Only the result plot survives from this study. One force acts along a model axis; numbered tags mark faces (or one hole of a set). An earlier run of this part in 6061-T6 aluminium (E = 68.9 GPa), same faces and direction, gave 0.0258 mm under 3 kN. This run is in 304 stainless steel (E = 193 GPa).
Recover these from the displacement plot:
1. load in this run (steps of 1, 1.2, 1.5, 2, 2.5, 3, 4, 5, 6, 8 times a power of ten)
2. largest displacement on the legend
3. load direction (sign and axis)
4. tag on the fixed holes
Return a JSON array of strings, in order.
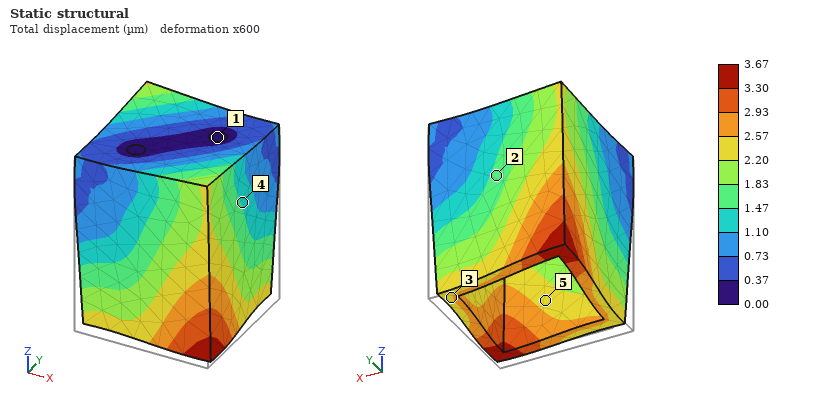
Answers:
["1.2 kN", "3.67 µm", "+Z", "1"]
